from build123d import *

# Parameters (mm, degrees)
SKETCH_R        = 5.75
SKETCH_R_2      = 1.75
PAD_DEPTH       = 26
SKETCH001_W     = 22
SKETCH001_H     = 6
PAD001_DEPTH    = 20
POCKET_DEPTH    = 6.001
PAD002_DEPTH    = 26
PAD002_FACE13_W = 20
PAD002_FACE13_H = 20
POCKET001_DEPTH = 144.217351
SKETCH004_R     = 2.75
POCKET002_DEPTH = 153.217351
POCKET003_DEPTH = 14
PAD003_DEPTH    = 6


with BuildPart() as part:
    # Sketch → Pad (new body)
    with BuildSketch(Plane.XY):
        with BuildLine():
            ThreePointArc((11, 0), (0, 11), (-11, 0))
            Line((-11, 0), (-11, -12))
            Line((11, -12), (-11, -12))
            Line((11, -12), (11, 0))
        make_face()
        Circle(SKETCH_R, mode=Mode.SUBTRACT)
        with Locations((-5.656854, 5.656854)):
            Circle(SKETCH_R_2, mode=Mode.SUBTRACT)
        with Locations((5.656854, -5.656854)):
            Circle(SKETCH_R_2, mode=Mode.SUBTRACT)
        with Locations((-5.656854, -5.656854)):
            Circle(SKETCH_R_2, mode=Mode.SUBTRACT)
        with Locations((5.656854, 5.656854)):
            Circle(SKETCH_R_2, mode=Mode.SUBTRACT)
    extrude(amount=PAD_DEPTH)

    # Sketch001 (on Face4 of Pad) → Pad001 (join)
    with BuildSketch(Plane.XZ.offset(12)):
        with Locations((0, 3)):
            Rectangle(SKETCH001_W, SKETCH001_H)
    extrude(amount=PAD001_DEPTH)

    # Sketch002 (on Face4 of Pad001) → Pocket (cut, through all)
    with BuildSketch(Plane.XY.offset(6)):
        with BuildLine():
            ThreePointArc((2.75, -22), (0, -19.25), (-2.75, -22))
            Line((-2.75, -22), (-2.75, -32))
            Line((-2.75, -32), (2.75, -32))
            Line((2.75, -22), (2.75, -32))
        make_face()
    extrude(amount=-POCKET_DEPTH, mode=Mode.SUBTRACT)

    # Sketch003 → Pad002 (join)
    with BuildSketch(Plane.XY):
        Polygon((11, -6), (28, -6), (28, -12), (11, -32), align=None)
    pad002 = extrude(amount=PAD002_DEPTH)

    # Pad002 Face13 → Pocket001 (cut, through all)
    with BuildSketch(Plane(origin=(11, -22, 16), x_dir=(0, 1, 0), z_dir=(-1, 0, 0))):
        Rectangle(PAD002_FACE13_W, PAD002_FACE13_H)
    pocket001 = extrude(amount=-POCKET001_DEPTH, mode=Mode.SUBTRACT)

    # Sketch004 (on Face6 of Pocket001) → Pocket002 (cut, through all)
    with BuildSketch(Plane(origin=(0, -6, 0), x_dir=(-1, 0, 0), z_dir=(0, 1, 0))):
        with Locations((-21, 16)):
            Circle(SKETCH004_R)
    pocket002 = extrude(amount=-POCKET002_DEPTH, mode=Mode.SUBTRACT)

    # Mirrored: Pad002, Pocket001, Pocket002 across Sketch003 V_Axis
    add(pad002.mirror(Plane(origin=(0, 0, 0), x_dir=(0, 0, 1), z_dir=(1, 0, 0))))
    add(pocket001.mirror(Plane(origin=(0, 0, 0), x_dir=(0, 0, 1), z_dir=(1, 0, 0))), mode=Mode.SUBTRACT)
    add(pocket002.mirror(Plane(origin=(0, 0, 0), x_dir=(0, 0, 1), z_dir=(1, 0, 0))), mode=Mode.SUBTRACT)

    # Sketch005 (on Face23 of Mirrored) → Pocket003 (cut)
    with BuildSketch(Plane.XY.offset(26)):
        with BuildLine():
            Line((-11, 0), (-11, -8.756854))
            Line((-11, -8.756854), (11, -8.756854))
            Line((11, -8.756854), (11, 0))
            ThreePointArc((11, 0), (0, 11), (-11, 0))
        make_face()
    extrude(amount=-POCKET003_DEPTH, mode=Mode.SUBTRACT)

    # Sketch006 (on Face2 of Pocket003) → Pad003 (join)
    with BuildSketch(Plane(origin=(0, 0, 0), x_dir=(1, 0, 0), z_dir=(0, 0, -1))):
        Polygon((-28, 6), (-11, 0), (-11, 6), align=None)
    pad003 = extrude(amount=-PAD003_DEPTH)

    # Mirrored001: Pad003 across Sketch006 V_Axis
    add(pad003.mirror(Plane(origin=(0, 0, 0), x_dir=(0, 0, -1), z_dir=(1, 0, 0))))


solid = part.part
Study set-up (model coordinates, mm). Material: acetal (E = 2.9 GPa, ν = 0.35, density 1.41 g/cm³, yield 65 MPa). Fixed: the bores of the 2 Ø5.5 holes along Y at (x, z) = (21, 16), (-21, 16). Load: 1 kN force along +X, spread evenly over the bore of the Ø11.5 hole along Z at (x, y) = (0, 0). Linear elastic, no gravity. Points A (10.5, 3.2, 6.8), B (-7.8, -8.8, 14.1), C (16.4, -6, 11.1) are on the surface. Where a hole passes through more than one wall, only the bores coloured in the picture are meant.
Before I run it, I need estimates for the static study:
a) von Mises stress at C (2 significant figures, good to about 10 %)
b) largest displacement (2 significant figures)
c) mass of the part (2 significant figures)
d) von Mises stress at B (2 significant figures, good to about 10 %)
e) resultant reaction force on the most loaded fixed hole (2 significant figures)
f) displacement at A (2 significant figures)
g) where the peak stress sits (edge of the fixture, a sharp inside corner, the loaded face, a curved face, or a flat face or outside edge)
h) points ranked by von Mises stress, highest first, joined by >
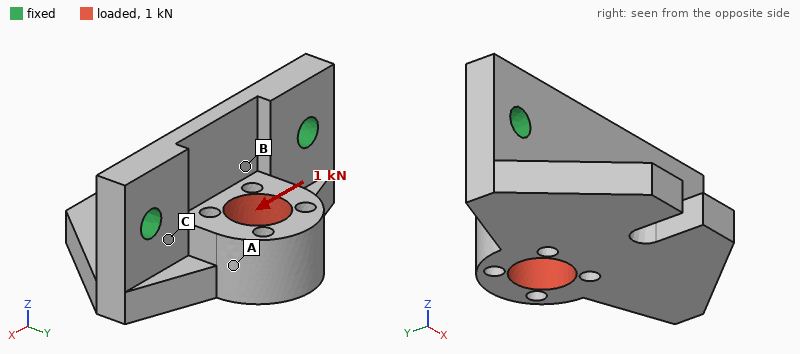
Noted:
12 MPa
0.25 mm
21 g
8.5 MPa
580 N
0.18 mm
a curved face
C > B > A
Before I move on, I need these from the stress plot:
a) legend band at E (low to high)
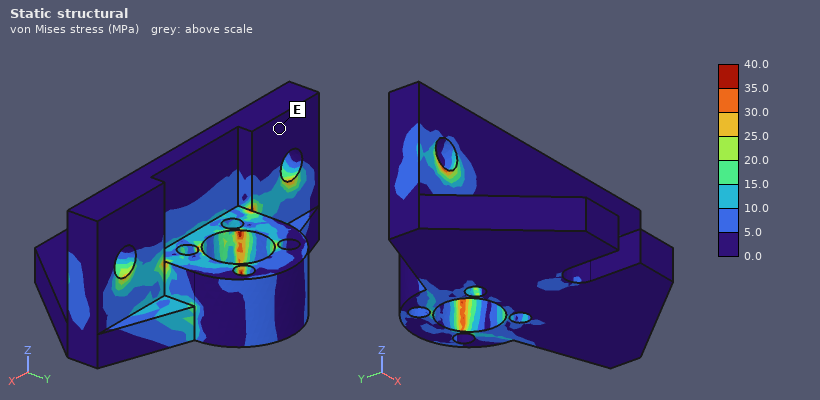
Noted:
0.0 to 5.0 MPa
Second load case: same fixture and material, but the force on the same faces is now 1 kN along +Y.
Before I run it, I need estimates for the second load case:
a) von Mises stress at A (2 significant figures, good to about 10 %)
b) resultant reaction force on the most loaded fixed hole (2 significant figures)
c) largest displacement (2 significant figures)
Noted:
7.4 MPa
500 N
0.70 mm
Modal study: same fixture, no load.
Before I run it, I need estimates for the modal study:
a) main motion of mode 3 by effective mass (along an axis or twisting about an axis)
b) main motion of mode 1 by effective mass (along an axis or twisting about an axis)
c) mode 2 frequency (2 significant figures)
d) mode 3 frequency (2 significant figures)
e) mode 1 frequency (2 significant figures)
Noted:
along Y
along Y
3100 Hz
3500 Hz
1500 Hz
